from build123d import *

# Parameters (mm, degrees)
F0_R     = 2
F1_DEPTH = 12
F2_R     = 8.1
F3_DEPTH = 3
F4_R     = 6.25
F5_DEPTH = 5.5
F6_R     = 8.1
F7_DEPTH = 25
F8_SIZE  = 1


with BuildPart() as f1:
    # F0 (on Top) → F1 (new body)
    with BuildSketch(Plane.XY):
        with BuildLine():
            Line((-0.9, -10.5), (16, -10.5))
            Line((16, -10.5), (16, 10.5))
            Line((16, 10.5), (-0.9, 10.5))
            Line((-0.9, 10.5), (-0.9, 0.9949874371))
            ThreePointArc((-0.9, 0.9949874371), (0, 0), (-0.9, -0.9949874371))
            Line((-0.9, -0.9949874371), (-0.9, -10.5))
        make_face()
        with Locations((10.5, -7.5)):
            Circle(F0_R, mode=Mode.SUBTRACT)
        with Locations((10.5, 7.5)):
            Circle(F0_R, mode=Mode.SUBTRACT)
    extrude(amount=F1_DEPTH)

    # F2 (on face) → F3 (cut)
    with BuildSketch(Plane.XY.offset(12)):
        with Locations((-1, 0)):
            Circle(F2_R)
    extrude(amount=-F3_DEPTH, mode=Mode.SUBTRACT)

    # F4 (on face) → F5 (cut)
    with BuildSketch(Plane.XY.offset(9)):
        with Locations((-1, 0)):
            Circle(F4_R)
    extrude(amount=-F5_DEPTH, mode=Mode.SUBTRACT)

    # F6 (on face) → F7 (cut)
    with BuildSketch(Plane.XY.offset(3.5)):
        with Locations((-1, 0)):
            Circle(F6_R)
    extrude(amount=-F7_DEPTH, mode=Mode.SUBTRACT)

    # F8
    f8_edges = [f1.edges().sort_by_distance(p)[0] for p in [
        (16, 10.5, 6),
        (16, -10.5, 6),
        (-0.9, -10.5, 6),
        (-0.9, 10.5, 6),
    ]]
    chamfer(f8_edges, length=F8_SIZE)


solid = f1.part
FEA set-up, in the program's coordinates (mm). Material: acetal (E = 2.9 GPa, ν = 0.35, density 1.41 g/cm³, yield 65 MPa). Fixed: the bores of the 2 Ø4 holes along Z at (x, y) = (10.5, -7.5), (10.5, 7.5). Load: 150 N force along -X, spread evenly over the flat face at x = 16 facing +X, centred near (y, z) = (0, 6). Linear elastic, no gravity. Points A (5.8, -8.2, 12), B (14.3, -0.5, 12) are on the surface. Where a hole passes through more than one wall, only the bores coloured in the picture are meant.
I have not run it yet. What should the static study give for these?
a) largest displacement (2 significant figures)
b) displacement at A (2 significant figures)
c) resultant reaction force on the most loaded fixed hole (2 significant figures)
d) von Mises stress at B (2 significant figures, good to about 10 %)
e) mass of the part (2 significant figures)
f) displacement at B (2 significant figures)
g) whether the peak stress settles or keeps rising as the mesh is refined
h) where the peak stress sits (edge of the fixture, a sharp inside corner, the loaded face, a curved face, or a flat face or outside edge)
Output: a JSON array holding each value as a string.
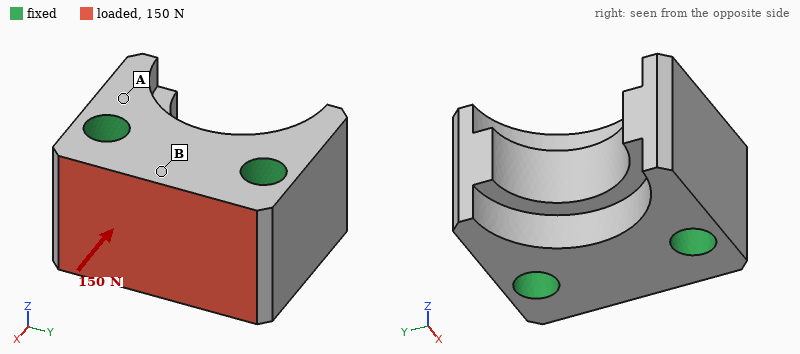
["2.8 µm", "0.44 µm", "77 N", "0.52 MPa", "4.1 g", "2.5 µm", "keeps rising", "edge of the fixture"]
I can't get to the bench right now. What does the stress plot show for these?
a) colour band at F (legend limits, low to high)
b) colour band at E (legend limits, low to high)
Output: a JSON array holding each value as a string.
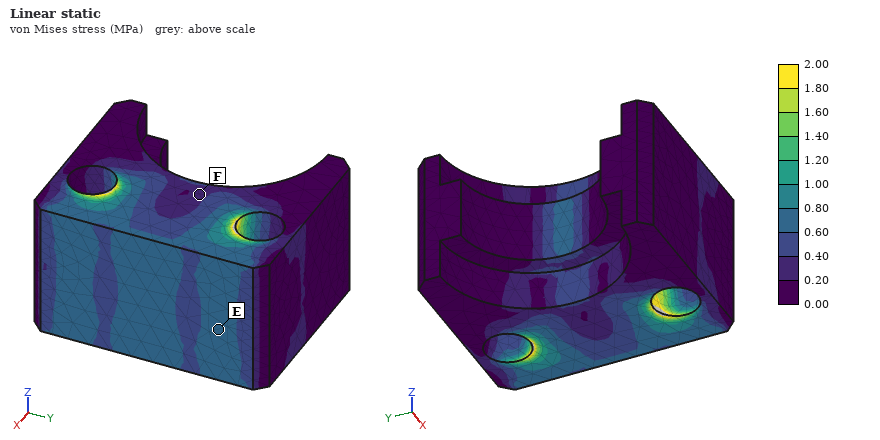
["0.20 to 0.40 MPa", "0.60 to 0.80 MPa"]
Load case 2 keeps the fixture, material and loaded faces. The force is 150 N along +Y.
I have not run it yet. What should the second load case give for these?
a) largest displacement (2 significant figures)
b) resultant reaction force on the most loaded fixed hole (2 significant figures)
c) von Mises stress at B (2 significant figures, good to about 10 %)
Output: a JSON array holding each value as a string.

["3.6 µm", "84 N", "1.1 MPa"]
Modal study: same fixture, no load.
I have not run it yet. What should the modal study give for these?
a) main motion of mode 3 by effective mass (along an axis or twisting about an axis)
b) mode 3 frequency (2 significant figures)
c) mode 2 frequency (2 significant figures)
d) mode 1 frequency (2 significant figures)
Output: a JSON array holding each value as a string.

["along Z", "20 kHz", "17 kHz", "17 kHz"]
